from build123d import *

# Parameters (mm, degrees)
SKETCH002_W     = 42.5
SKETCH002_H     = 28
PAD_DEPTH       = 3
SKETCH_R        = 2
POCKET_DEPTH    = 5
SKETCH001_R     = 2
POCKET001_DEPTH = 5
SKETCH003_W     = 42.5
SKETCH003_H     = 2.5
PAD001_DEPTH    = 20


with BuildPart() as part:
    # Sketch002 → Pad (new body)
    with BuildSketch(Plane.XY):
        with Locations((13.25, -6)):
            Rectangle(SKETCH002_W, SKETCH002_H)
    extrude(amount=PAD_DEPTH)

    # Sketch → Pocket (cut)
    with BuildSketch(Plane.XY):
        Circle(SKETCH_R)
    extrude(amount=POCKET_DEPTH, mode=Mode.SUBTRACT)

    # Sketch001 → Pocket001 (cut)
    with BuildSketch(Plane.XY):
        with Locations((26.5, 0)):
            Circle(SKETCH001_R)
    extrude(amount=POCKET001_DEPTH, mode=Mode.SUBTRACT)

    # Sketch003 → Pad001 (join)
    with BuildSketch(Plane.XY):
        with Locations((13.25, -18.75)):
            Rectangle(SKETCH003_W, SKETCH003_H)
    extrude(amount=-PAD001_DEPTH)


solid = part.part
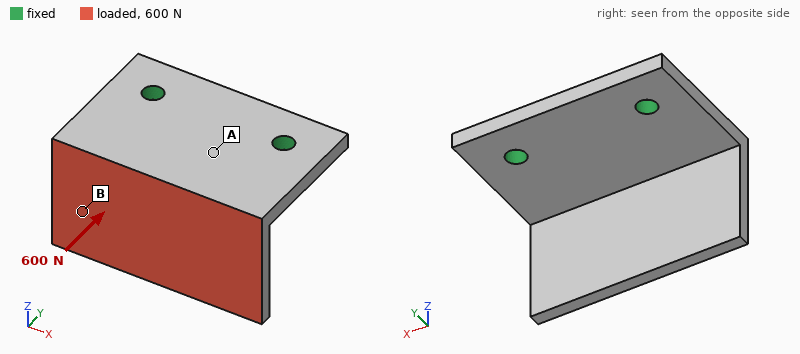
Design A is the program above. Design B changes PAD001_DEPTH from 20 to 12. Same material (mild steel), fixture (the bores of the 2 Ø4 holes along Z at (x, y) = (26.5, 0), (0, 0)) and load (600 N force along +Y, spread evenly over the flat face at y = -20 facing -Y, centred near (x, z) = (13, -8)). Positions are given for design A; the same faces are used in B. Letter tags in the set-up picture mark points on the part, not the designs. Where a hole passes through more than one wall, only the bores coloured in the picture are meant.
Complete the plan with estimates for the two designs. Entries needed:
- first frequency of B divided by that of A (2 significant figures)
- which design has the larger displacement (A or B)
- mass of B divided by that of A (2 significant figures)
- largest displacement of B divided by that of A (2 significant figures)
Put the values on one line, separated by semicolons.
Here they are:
1.5; A; 0.85; 0.37
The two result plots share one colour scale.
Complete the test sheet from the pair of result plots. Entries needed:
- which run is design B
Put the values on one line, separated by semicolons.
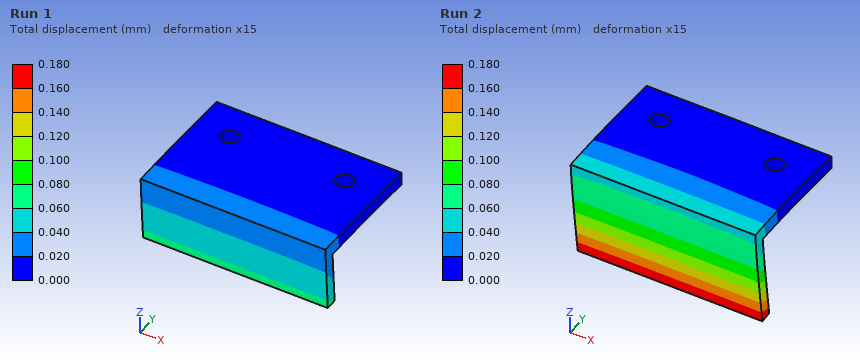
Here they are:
Run 1
